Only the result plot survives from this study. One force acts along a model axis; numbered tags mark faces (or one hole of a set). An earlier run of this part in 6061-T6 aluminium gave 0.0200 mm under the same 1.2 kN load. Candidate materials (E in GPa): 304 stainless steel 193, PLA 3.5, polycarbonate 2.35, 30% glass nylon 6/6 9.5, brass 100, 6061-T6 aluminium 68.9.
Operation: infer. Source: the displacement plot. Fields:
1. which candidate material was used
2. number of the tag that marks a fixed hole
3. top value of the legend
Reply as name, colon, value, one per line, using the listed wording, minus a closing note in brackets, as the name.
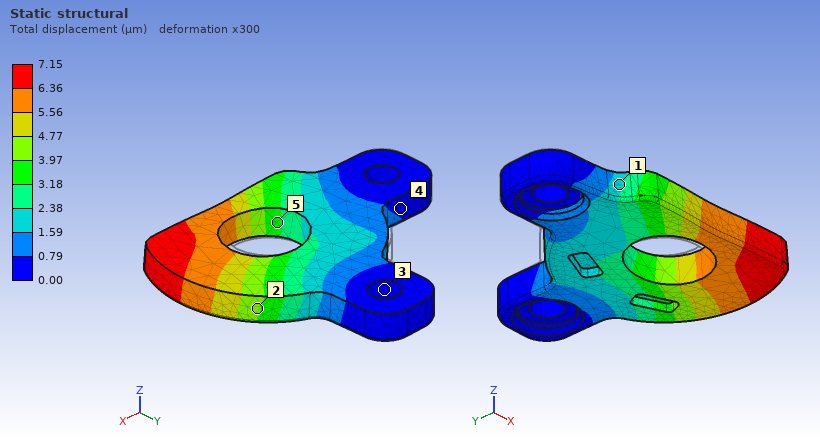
which candidate material was used: 304 stainless steel
number of the tag that marks a fixed hole: 3
top value of the legend: 7.15 µm
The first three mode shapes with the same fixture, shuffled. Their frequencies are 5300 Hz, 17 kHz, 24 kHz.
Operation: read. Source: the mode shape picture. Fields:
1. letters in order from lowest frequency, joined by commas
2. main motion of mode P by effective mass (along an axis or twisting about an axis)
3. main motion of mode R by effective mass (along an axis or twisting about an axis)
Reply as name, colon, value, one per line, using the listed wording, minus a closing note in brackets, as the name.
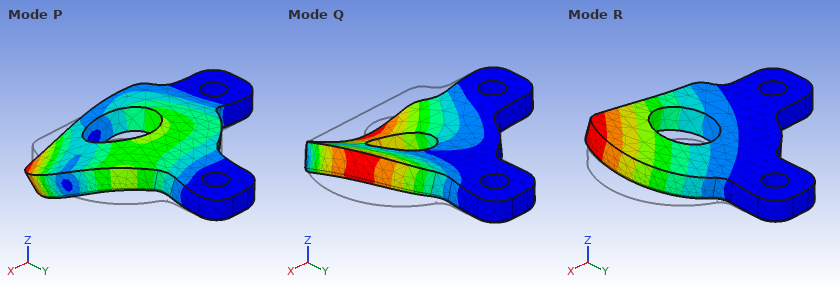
letters in order from lowest frequency, joined by commas: R, Q, P
main motion of mode P by effective mass: along Z
main motion of mode R by effective mass: along Z
